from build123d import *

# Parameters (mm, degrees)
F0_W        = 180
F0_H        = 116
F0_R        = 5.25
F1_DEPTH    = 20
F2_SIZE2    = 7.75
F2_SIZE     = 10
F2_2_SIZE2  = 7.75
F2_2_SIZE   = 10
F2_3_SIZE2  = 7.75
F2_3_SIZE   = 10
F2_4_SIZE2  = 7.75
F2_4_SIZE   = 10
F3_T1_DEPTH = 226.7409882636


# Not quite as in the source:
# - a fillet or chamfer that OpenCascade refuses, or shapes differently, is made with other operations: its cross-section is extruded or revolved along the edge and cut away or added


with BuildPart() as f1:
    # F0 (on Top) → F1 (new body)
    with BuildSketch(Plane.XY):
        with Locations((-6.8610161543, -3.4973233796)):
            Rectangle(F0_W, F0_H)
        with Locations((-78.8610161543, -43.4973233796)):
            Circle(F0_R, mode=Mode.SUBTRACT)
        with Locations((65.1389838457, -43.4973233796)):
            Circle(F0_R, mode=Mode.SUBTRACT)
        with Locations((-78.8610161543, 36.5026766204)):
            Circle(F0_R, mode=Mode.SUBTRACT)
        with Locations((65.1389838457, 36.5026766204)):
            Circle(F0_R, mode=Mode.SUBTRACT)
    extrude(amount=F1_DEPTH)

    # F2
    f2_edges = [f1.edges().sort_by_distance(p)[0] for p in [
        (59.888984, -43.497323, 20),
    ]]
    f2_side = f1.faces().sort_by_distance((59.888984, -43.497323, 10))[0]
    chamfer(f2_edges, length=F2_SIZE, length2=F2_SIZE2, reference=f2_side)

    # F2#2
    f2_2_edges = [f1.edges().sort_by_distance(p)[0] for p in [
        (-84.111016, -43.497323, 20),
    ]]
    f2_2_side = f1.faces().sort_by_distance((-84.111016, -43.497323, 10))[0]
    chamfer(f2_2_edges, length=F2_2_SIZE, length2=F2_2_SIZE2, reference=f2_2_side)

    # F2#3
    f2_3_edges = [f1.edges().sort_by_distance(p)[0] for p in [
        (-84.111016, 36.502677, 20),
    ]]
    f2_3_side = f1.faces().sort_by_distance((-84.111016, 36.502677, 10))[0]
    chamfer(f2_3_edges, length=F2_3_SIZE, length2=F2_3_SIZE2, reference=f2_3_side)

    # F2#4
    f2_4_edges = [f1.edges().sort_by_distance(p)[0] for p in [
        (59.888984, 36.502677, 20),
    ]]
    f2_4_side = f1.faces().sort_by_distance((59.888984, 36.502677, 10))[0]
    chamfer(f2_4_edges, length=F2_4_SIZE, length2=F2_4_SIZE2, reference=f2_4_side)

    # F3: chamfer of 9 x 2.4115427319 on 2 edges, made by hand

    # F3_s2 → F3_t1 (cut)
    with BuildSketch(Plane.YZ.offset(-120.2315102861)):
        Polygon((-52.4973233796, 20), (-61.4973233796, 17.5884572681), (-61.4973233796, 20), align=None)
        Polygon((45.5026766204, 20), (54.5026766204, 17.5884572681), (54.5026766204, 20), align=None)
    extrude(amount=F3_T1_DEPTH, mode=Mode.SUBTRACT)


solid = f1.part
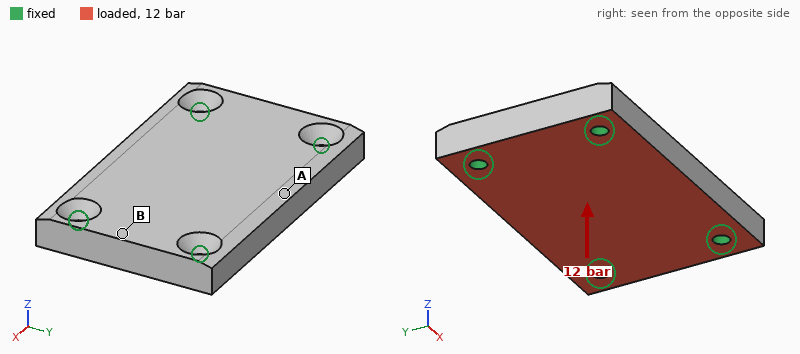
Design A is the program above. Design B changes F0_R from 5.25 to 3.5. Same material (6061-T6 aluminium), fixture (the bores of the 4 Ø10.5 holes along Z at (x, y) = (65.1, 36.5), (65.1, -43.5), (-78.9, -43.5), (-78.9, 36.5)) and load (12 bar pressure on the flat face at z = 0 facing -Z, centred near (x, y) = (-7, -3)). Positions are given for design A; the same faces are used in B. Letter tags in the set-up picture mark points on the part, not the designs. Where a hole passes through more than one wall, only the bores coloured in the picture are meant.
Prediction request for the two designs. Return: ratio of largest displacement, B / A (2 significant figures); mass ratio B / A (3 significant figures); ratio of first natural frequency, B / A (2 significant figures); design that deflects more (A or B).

1.2
1.01
0.92
B
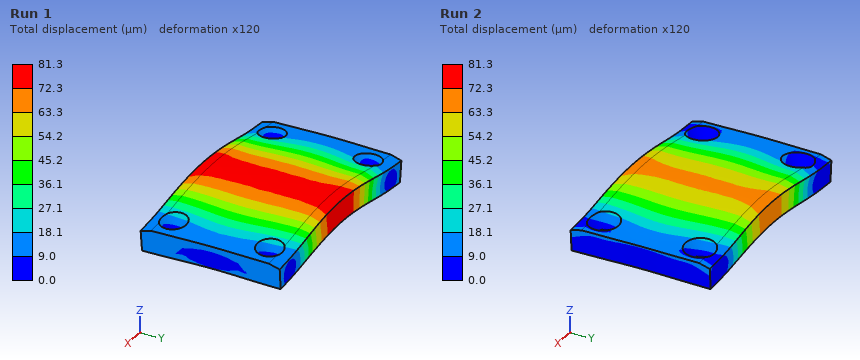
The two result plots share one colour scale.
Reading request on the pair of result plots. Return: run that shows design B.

Run 1
